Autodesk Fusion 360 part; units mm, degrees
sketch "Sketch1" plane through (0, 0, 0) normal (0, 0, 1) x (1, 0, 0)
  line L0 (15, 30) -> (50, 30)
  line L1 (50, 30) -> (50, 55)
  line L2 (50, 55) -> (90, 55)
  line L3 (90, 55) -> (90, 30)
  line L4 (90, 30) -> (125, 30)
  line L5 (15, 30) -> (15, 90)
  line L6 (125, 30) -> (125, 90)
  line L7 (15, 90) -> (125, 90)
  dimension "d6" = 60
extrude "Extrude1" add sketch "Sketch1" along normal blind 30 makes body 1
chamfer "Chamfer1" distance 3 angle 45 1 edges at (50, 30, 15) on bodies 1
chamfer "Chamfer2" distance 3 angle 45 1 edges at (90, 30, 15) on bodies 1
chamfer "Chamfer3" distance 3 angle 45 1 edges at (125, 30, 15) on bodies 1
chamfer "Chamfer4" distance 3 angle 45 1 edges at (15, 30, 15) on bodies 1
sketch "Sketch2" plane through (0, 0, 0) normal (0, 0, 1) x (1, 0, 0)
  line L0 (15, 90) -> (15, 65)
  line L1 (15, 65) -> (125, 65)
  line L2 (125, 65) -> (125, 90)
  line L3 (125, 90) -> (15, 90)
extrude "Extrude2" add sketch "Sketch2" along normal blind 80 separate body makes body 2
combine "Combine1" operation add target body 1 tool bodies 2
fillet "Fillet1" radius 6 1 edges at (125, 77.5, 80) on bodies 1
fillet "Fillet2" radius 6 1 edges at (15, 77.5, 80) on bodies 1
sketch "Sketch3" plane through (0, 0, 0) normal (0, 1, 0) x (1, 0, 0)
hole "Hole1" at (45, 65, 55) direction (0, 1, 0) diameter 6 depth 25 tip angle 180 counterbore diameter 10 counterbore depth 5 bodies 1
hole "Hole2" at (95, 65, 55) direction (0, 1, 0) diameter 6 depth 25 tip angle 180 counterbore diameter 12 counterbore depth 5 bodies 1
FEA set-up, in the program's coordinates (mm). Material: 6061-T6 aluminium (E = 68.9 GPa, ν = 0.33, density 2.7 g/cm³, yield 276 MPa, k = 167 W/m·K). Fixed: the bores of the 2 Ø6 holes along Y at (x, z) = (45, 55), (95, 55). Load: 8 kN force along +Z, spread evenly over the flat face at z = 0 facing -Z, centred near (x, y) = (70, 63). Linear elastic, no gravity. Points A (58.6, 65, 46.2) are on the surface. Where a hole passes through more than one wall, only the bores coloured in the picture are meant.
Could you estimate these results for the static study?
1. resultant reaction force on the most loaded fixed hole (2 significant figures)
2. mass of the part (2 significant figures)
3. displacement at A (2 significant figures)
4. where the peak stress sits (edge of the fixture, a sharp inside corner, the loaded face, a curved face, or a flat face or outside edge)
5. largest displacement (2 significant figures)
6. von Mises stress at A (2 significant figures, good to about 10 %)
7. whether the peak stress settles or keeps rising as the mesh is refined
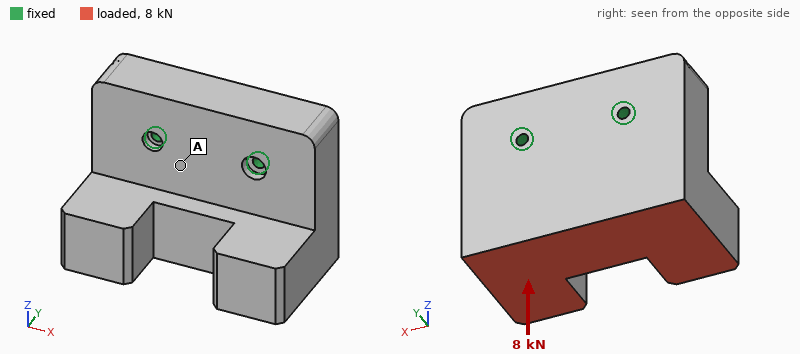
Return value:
4.0 kN
820 g
8.7 µm
edge of the fixture
54 µm
9.4 MPa
keeps rising
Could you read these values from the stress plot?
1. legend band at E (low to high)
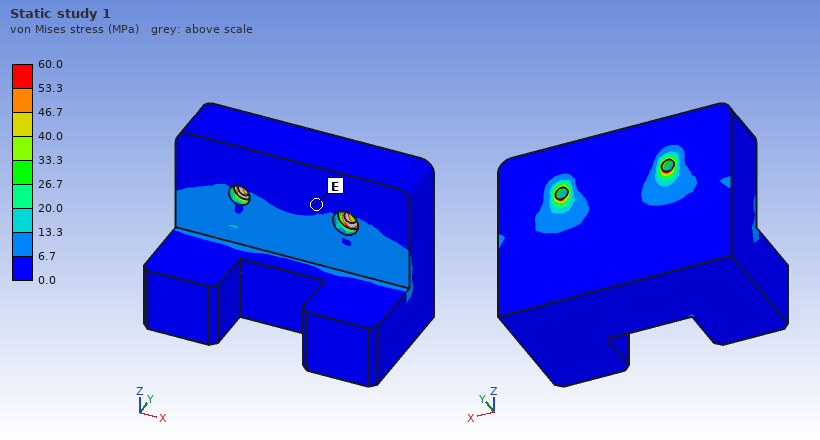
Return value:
0.0 to 6.7 MPa
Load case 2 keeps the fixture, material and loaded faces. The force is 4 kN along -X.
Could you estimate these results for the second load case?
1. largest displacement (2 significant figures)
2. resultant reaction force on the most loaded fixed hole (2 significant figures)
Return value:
16 µm
4.7 kN
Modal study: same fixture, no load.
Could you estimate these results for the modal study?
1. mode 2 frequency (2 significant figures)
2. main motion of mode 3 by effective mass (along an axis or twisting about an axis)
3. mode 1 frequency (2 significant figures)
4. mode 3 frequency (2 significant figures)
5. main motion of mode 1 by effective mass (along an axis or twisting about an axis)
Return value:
3800 Hz
along X
2300 Hz
5100 Hz
along Y
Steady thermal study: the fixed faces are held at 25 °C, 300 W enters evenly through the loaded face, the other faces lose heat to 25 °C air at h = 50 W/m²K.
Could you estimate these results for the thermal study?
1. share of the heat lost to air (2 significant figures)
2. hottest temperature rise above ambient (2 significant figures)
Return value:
10 %
40 K
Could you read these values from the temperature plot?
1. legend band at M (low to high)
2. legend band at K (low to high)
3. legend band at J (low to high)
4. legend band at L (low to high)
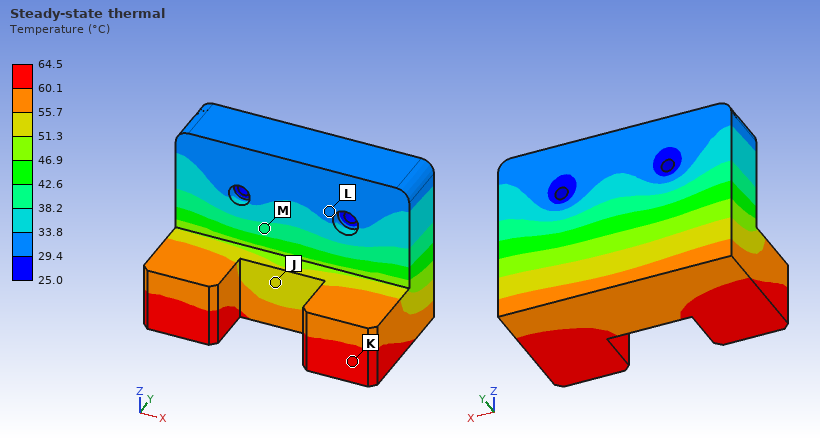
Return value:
38.2 to 42.6 °C
60.1 to 64.5 °C
51.3 to 55.7 °C
29.4 to 33.8 °C
